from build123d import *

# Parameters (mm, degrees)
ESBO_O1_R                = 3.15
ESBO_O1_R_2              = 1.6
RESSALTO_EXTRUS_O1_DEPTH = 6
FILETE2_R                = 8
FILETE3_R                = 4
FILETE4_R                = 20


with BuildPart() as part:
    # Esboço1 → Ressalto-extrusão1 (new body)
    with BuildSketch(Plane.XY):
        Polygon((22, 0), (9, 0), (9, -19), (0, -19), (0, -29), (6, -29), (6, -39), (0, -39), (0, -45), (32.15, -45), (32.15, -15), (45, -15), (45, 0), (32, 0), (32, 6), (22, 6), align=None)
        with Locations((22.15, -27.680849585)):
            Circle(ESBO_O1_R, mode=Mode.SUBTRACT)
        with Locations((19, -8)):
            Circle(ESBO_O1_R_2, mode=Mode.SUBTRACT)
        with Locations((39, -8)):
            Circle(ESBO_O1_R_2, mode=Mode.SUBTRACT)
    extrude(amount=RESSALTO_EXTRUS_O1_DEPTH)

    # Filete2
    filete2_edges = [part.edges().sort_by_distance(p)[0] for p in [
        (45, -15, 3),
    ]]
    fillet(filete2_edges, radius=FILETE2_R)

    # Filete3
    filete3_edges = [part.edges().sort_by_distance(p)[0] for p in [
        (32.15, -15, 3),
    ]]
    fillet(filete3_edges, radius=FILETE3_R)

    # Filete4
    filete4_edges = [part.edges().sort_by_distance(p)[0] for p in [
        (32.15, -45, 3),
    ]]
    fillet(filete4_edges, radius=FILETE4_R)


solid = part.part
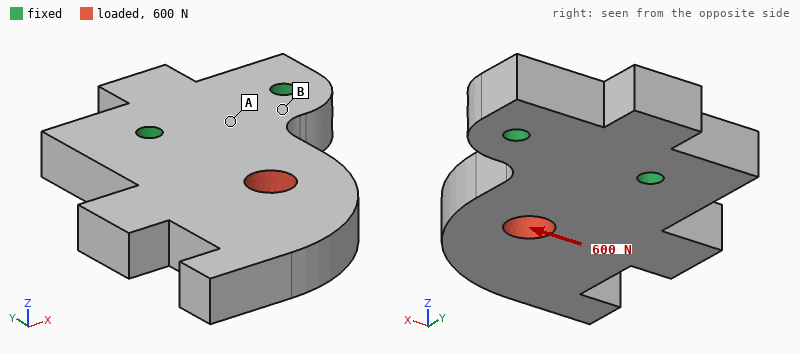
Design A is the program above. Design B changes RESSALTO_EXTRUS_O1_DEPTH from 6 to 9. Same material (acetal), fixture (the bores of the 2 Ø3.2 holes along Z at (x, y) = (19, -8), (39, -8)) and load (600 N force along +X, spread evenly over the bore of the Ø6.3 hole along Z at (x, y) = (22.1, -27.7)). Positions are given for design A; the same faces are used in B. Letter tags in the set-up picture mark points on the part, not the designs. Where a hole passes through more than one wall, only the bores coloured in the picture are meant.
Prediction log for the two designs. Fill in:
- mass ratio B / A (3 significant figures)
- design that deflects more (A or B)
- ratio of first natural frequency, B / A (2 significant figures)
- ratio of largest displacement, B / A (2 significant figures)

1.50
A
1.4
0.66
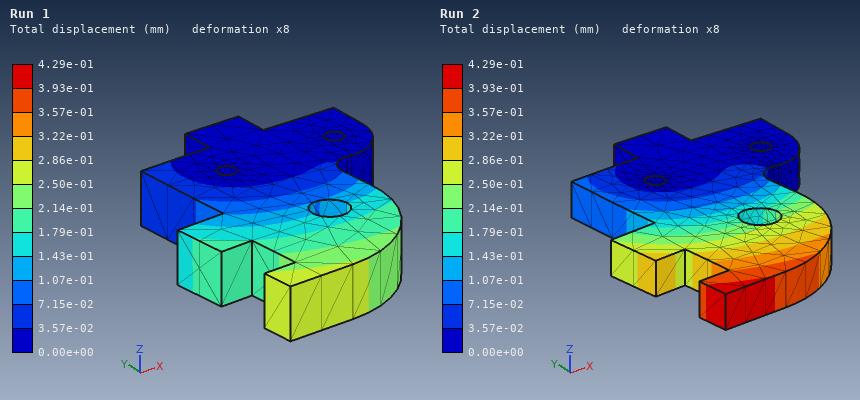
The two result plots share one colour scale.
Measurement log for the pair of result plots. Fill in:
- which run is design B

Run 1
